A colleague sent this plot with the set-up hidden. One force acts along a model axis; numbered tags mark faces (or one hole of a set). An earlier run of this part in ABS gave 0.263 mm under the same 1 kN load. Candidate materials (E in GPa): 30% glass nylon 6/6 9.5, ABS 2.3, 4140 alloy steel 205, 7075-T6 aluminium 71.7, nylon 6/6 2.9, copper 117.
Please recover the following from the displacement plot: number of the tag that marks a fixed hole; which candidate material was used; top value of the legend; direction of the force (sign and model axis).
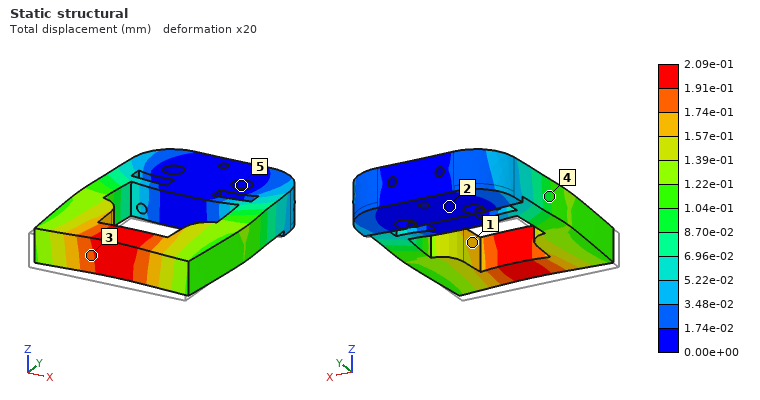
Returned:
5
nylon 6/6
2.09e-01 mm
+Y
